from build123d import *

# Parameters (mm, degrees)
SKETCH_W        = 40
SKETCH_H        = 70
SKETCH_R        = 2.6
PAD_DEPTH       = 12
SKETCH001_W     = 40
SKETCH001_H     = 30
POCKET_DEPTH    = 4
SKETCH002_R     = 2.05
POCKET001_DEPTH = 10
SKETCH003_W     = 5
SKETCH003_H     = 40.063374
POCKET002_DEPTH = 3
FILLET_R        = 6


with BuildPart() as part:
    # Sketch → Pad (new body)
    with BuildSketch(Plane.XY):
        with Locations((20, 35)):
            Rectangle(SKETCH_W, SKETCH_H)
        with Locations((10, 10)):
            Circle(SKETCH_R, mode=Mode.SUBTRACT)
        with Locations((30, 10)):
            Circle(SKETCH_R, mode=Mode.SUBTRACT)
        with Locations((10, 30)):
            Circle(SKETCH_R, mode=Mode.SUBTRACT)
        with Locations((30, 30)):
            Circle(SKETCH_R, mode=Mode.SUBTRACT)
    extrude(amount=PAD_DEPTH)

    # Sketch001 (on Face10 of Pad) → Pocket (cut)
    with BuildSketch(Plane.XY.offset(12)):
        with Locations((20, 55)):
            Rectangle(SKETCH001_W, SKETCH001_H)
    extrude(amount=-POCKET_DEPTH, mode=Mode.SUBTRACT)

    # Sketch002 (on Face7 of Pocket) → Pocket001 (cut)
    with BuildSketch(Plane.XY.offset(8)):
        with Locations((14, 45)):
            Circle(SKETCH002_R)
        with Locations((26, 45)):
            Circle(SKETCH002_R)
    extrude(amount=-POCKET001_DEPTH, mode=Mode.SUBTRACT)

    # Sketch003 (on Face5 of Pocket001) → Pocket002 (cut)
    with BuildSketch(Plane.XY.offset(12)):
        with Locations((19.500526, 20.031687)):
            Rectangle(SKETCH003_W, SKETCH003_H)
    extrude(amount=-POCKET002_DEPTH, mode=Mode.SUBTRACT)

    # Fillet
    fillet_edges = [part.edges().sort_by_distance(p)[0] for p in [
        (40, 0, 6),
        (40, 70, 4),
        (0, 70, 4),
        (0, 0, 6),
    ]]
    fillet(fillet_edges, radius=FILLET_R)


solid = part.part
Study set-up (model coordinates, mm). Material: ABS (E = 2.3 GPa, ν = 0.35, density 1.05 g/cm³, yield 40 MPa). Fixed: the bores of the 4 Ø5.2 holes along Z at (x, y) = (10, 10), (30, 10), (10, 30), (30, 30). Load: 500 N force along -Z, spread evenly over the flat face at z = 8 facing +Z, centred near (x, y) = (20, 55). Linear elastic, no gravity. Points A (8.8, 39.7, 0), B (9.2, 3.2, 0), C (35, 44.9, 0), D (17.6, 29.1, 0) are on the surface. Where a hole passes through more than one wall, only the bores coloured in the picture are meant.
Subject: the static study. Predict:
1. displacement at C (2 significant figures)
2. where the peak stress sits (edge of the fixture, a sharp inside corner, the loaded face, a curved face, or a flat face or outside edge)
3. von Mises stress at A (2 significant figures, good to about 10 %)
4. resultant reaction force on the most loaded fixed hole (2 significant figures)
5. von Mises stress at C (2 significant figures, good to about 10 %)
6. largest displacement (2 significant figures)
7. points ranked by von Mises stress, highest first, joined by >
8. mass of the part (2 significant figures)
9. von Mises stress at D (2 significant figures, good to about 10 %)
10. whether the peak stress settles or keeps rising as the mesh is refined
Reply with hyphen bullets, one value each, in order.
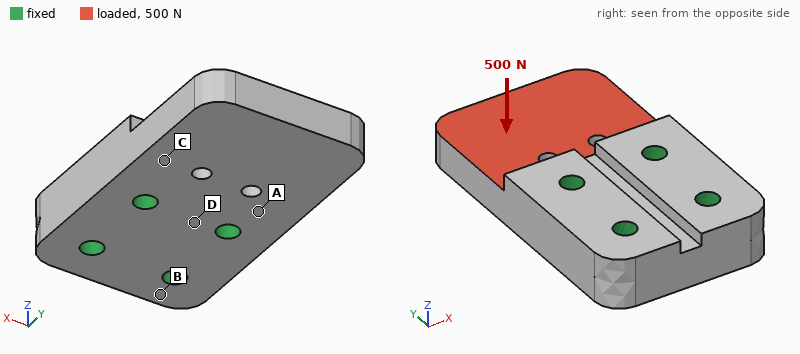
- 0.17 mm
- edge of the fixture
- 16 MPa
- 310 N
- 13 MPa
- 0.92 mm
- A > C > D > B
- 28 g
- 5.7 MPa
- keeps rising
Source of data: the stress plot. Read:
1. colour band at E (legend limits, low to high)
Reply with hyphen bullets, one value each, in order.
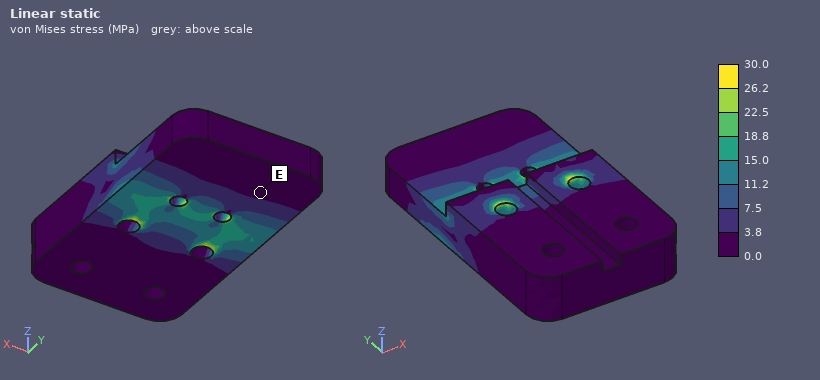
- 0.0 to 3.8 MPa
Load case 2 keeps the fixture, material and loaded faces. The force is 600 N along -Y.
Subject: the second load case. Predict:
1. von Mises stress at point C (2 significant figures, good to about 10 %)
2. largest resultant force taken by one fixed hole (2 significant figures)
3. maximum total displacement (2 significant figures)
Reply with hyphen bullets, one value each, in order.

- 3.5 MPa
- 260 N
- 0.28 mm
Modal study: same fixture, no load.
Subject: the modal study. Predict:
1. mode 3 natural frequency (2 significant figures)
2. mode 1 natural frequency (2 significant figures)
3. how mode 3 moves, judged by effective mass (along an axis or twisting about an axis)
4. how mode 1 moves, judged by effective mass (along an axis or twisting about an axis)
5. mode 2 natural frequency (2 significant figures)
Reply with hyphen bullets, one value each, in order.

- 3700 Hz
- 1500 Hz
- along X
- along Z
- 3000 Hz
